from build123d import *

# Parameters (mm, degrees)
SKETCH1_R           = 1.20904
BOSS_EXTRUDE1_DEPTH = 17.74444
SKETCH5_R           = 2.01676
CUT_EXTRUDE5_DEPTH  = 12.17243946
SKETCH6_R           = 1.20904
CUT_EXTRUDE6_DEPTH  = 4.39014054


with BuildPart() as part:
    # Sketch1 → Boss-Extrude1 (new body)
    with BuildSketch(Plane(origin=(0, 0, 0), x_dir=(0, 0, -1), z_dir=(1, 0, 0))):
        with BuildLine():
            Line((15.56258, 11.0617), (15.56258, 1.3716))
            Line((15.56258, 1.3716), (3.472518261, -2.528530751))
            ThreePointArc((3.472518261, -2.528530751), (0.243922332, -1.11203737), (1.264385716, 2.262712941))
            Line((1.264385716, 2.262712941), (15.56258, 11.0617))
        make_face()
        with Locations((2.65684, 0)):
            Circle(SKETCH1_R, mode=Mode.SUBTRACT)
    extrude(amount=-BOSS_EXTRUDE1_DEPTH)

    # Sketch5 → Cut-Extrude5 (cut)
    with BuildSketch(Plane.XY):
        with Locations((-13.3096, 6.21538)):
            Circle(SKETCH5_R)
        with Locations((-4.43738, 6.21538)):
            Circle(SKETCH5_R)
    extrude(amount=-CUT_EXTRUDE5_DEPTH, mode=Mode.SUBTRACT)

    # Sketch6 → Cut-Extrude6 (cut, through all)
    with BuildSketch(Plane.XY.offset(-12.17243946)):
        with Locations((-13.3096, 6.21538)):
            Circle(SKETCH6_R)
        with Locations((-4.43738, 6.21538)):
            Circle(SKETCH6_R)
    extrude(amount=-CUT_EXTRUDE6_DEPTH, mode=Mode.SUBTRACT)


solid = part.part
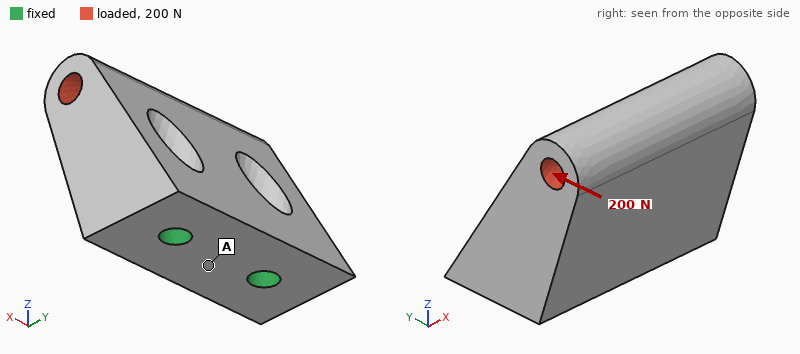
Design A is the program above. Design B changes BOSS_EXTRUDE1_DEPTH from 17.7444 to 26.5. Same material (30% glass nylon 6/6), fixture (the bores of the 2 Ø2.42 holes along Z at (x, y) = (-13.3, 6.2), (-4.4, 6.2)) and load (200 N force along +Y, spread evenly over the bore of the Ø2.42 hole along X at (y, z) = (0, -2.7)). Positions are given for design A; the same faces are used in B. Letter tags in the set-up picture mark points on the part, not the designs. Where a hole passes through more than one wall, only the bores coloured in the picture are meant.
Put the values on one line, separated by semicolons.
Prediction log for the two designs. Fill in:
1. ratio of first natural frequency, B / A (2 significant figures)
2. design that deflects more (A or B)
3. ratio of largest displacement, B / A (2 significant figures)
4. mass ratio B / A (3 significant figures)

0.75; B; 1.2; 1.53
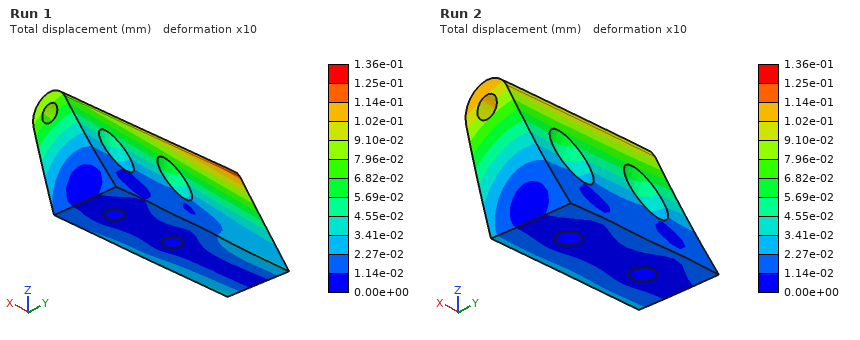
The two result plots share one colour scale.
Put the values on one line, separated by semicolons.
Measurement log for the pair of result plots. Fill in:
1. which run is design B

Run 1
